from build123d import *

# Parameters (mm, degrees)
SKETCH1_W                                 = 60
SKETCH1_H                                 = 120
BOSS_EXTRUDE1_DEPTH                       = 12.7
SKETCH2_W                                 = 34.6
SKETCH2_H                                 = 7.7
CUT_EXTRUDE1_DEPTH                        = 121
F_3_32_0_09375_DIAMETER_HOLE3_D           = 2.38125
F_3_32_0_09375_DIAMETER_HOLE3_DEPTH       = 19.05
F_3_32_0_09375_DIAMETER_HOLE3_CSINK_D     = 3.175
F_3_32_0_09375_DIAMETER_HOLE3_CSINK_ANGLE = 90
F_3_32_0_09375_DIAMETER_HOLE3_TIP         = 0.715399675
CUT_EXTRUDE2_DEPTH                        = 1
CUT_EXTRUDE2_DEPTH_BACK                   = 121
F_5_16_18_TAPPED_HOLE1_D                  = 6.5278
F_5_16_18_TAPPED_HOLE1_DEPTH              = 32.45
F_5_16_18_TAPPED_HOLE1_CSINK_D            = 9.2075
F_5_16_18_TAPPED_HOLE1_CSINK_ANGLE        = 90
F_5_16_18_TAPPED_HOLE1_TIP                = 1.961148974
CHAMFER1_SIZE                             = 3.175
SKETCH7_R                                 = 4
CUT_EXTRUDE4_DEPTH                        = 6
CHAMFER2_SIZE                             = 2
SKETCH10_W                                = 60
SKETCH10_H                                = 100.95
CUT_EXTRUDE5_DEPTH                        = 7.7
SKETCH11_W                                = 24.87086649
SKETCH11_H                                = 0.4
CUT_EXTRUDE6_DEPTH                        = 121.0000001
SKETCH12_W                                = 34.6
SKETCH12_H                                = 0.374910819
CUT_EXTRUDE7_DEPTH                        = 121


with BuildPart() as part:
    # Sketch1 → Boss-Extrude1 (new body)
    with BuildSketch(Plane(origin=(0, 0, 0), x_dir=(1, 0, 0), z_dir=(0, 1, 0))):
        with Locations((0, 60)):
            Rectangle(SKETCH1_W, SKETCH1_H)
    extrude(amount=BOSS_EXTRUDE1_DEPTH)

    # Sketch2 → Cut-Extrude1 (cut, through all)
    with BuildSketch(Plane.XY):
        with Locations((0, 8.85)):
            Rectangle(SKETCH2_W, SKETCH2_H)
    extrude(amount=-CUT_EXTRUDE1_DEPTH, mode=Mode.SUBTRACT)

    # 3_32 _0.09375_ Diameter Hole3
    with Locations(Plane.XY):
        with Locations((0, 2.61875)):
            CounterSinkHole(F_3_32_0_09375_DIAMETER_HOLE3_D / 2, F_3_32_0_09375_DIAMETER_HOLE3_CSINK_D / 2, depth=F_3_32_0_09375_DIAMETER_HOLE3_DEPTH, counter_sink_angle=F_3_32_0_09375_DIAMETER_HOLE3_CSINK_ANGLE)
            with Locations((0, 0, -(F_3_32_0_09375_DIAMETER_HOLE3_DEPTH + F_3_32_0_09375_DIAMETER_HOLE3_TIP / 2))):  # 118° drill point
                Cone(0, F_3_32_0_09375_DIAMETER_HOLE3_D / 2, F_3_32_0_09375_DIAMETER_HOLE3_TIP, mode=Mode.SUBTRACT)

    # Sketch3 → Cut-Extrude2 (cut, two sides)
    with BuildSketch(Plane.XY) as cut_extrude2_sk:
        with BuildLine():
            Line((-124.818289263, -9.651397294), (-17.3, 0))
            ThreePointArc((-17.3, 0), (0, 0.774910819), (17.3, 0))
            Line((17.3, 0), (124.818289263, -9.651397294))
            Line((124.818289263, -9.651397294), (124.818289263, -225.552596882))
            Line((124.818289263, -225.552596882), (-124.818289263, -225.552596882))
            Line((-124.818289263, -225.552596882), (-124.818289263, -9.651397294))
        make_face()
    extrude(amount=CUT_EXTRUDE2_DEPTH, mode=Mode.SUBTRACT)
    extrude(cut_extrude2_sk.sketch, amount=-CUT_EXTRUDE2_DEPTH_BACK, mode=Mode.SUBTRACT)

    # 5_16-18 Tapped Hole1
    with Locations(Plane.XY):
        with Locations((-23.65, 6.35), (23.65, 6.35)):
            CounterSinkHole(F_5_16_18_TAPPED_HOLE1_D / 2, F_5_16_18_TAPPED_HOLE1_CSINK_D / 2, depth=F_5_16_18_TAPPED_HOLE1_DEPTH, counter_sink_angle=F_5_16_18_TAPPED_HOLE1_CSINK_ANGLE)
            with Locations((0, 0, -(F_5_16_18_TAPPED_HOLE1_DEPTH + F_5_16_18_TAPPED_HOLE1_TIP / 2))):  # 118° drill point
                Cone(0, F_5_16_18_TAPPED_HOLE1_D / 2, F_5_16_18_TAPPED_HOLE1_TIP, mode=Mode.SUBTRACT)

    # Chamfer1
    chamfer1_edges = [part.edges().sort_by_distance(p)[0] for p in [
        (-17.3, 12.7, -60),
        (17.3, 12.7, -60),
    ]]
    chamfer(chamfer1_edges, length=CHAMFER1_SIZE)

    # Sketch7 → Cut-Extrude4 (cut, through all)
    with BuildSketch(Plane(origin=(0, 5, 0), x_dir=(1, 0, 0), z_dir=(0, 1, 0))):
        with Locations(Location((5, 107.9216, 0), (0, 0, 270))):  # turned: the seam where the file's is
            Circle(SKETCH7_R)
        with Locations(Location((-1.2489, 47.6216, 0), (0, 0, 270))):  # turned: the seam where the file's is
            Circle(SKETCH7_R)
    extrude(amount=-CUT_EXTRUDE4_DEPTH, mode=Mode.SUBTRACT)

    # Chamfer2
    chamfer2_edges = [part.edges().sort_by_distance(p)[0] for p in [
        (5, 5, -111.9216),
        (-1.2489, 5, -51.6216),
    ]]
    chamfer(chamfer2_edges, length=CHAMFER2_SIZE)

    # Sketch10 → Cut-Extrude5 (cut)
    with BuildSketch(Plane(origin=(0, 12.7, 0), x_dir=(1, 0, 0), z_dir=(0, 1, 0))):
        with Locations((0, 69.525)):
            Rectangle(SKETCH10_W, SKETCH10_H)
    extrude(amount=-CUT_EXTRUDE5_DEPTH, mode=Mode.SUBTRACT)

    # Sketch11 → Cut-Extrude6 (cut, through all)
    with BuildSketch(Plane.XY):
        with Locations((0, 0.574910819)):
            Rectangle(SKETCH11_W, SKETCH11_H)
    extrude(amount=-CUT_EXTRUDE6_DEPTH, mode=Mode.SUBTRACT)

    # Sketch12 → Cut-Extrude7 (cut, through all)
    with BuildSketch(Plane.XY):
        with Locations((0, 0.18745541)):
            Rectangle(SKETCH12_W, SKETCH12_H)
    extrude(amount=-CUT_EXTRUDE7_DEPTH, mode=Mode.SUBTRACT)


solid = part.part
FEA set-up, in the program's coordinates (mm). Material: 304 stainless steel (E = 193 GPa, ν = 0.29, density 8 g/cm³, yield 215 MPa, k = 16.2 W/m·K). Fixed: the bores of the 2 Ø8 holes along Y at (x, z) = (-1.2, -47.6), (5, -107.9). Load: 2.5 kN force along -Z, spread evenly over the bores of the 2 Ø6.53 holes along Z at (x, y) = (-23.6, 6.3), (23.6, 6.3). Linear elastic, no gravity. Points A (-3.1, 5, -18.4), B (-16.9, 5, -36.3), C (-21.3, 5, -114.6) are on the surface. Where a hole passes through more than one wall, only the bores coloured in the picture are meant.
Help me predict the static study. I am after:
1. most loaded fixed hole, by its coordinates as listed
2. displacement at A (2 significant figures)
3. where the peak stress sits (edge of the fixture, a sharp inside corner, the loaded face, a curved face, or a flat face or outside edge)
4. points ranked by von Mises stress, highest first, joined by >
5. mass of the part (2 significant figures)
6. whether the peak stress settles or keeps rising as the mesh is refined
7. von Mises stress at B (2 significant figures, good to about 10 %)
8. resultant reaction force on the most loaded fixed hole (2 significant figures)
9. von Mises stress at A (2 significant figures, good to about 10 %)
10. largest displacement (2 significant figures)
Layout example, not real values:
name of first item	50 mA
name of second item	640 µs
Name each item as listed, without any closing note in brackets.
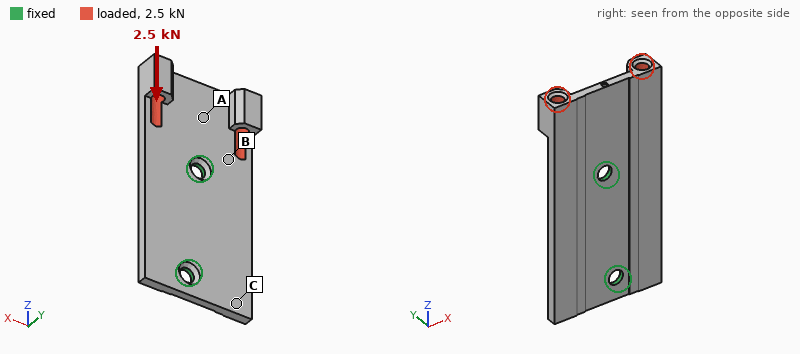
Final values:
most loaded fixed hole, by its coordinates as listed	(-1.2, -47.6)
displacement at A	0.050 mm
where the peak stress sits	edge of the fixture
points ranked by von Mises stress, highest first, joined by >	B > A > C
mass of the part	280 g
whether the peak stress settles or keeps rising as the mesh is refined	keeps rising
von Mises stress at B	43 MPa
resultant reaction force on the most loaded fixed hole	1.8 kN
von Mises stress at A	27 MPa
largest displacement	0.12 mm
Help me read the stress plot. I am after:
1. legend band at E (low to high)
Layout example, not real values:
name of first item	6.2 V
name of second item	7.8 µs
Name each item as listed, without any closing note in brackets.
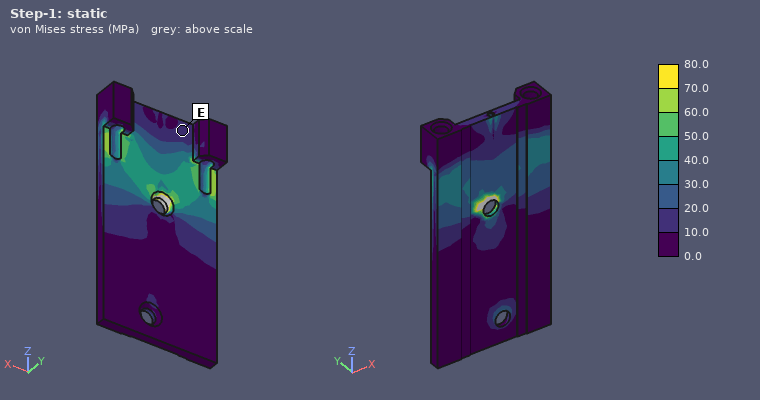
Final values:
legend band at E	10.0 to 20.0 MPa
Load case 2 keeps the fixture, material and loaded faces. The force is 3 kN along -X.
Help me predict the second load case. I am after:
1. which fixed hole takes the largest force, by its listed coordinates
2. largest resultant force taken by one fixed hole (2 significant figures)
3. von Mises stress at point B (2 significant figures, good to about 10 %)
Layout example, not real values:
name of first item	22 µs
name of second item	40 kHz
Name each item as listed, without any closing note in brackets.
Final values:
which fixed hole takes the largest force, by its listed coordinates	(-1.2, -47.6)
largest resultant force taken by one fixed hole	4.4 kN
von Mises stress at point B	46 MPa
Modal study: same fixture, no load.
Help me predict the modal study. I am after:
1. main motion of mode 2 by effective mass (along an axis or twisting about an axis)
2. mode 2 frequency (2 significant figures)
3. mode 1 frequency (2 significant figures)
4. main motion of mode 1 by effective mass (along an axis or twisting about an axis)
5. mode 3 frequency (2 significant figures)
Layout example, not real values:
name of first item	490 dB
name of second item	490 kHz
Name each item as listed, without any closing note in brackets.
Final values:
main motion of mode 2 by effective mass	twisting about Z
mode 2 frequency	1500 Hz
mode 1 frequency	1100 Hz
main motion of mode 1 by effective mass	along Y
mode 3 frequency	2500 Hz
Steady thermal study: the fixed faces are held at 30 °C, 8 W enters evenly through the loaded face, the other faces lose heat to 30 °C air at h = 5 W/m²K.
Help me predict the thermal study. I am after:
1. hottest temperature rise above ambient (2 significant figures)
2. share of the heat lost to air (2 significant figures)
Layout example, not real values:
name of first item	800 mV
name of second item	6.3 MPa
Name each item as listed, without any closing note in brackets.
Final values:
hottest temperature rise above ambient	71 K
share of the heat lost to air	26 %
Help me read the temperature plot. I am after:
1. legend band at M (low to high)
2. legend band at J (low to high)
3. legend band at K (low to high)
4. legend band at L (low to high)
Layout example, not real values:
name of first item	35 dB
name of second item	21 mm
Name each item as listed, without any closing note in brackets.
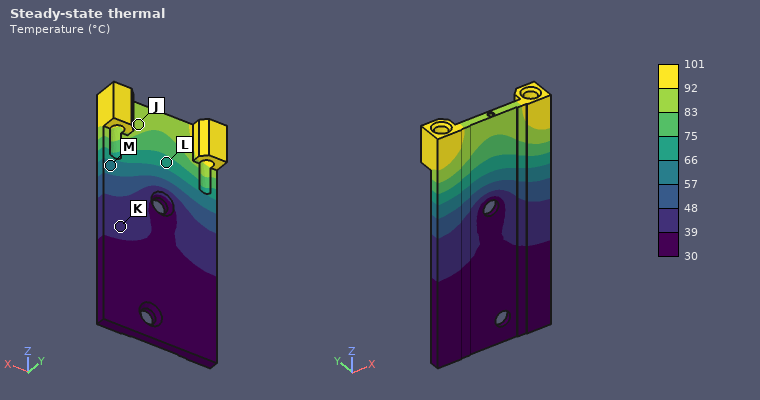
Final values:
legend band at M	57 to 66 °C
legend band at J	83 to 92 °C
legend band at K	39 to 48 °C
legend band at L	66 to 75 °C
